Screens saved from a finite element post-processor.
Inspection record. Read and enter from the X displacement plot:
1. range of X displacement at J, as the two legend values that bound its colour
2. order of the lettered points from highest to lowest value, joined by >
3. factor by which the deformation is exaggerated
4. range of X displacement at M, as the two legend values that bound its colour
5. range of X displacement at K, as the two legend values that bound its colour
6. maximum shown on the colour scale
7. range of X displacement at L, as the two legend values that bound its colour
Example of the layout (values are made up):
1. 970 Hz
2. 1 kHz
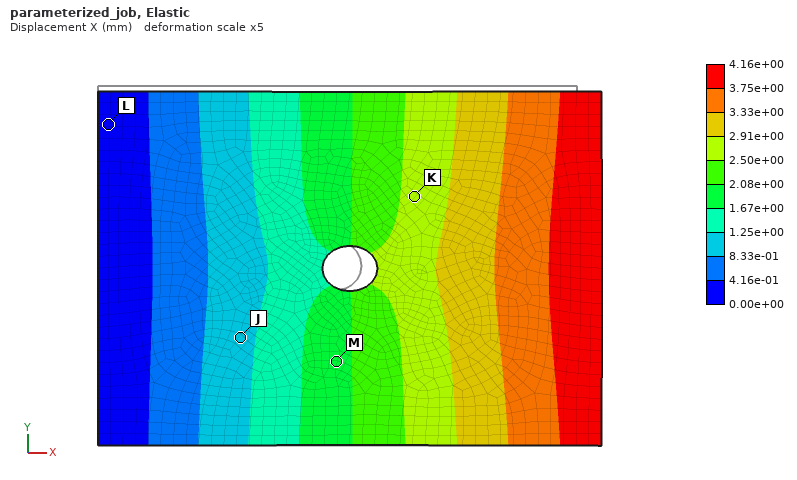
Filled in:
1. 8.33e-01 to 1.25e+00 mm
2. K > M > J > L
3. 5
4. 1.67e+00 to 2.08e+00 mm
5. 2.50e+00 to 2.91e+00 mm
6. 4.16e+00 mm
7. 0.00e+00 to 4.16e-01 mm
